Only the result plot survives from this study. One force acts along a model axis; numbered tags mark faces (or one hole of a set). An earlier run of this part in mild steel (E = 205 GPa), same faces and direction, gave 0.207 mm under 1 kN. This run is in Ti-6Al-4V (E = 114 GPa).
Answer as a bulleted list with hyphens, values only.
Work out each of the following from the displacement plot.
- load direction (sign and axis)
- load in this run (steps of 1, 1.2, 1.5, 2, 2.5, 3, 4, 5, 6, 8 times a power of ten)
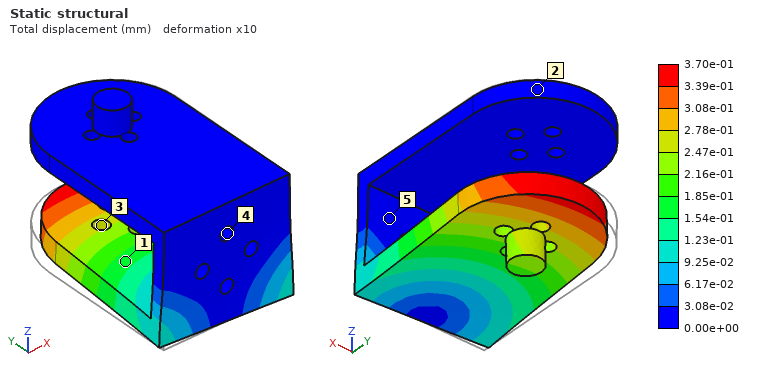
- +X
- 1 kN
